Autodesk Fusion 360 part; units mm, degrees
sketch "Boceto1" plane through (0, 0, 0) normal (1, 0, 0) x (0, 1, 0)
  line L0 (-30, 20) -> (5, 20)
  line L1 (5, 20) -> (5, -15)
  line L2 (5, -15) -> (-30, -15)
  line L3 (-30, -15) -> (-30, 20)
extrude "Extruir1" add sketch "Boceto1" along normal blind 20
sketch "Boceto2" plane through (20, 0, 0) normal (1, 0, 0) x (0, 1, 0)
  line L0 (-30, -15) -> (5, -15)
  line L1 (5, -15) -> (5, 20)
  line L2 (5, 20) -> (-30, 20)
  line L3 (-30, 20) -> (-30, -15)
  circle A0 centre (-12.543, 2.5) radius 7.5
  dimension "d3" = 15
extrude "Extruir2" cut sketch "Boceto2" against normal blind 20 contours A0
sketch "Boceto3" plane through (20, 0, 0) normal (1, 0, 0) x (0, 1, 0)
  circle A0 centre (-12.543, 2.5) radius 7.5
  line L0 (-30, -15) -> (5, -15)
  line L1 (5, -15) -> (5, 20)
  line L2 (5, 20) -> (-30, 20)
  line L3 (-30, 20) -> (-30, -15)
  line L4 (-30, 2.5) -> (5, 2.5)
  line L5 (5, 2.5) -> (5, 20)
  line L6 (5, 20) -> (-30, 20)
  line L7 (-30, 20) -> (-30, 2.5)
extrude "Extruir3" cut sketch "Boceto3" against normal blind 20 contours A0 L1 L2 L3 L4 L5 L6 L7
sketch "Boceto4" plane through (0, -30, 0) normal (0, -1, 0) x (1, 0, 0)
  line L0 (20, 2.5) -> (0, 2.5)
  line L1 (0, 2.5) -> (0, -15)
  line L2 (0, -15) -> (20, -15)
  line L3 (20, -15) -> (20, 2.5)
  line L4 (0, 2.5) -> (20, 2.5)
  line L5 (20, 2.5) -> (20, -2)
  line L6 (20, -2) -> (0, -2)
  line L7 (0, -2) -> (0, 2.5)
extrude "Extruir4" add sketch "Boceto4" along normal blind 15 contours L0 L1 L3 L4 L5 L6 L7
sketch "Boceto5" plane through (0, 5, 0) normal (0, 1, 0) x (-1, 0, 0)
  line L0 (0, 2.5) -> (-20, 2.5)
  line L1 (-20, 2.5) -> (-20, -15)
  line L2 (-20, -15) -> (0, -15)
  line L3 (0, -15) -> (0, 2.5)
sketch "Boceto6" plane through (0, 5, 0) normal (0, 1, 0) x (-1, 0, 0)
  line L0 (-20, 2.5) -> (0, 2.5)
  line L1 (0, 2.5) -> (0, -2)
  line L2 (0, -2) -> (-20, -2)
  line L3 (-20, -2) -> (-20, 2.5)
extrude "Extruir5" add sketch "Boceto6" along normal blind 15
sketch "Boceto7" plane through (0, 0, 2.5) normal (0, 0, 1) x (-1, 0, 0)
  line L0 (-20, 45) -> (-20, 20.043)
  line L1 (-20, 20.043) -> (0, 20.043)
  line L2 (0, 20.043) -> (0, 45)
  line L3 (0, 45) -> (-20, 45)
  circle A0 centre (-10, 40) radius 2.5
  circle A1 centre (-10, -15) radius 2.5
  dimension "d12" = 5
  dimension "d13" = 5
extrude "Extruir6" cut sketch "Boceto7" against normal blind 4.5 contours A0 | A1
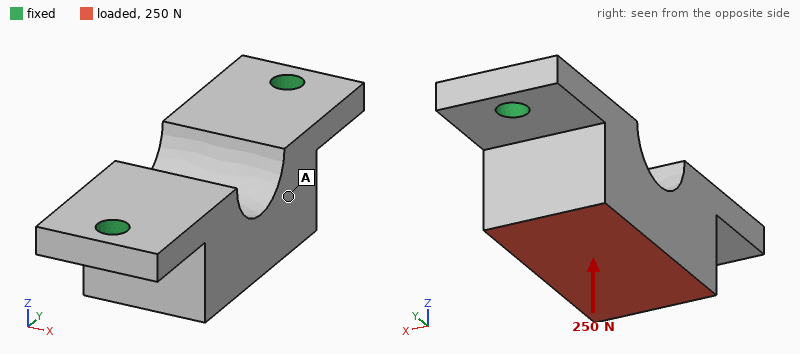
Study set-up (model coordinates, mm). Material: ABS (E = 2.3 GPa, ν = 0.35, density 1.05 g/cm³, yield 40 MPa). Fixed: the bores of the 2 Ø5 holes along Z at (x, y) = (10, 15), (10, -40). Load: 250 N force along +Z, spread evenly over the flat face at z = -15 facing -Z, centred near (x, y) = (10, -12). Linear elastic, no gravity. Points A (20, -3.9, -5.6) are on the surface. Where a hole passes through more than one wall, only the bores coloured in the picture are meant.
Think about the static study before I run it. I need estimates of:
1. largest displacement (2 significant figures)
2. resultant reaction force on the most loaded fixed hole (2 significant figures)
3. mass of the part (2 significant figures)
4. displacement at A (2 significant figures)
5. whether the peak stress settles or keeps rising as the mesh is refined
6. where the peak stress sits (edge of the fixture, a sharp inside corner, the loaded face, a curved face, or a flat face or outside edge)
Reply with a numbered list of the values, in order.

1. 91 µm
2. 170 N
3. 14 g
4. 85 µm
5. keeps rising
6. edge of the fixture
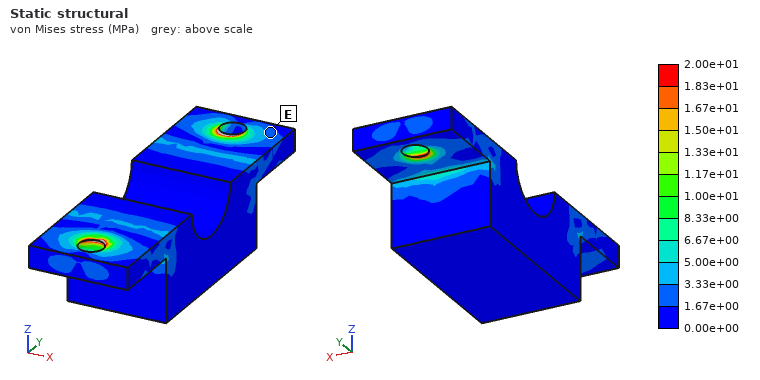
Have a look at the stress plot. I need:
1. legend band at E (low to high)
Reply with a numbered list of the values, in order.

1. 1.67e+00 to 3.33e+00 MPa
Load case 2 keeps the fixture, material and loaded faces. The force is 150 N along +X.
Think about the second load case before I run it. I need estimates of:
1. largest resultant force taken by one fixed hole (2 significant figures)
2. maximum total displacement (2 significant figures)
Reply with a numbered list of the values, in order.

1. 75 N
2. 0.42 mm
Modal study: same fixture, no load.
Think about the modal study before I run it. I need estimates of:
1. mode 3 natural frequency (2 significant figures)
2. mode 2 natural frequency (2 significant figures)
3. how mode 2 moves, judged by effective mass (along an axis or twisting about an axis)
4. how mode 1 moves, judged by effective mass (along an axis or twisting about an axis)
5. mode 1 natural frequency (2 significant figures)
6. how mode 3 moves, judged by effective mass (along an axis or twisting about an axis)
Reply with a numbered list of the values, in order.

1. 4100 Hz
2. 2600 Hz
3. along Z
4. along X
5. 1400 Hz
6. along Y
